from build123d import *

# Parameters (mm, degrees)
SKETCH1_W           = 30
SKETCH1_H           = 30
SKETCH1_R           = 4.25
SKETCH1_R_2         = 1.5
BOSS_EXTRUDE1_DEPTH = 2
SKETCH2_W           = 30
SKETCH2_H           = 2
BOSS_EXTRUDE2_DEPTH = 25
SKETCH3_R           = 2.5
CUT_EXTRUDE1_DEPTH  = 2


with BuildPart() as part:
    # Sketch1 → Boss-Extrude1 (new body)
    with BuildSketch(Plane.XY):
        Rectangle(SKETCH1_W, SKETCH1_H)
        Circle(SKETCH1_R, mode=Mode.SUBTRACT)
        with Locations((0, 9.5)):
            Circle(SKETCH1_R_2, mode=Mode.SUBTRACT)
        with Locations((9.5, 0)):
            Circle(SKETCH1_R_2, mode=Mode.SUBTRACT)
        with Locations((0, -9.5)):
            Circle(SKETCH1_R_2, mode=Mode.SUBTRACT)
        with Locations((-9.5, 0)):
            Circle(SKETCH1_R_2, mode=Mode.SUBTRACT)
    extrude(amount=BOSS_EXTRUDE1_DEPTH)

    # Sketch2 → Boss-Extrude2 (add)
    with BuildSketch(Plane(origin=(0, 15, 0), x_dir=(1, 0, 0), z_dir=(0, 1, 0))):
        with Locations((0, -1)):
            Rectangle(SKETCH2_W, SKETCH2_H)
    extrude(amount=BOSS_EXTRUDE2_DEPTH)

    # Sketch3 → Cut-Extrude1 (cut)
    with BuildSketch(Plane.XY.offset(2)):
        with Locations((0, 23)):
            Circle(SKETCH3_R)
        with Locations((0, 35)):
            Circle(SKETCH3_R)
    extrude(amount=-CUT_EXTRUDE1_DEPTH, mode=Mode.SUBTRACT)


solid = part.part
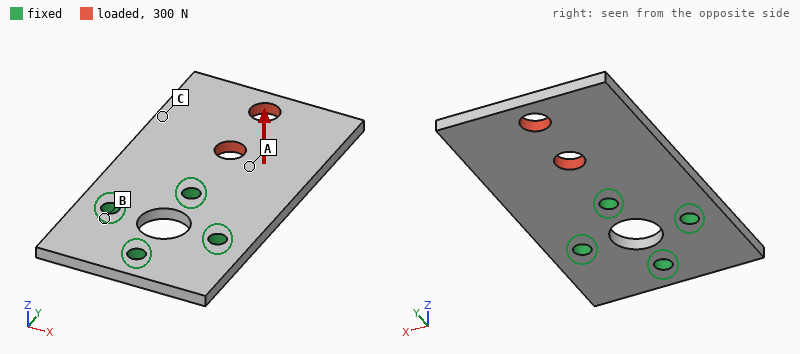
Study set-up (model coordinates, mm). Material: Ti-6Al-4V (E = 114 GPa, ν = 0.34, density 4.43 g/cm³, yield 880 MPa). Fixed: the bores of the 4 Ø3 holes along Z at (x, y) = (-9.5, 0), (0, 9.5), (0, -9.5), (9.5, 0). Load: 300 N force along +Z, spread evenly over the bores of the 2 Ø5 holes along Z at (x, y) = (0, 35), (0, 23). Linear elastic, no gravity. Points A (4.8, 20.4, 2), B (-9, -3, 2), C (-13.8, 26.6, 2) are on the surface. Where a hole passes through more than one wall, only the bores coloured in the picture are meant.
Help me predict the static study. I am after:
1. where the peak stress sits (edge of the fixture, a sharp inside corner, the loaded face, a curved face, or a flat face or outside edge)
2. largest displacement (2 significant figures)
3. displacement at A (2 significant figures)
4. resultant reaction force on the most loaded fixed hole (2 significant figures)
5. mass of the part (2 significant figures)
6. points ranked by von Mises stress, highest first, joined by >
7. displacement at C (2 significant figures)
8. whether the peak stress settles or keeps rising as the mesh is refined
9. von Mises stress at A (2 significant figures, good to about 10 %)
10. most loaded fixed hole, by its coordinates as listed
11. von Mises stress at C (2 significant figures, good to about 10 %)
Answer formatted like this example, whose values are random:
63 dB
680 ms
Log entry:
edge of the fixture
0.70 mm
0.15 mm
560 N
14 g
A > C > B
0.28 mm
keeps rising
140 MPa
(0, 9.5)
79 MPa
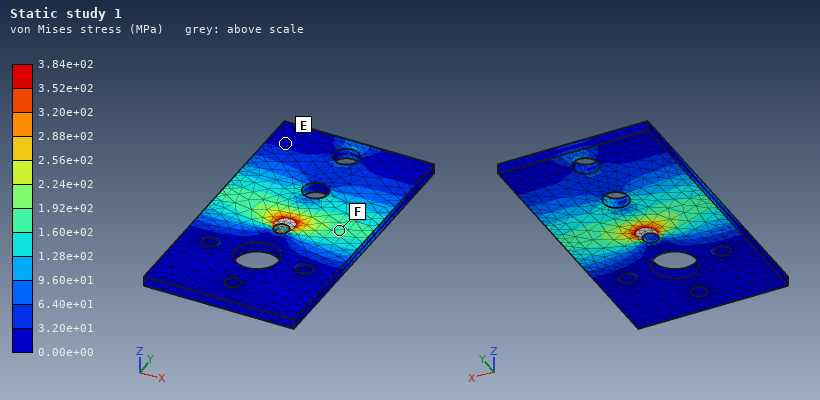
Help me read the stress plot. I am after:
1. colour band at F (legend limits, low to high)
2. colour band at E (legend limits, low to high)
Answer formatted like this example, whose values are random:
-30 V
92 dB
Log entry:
1.60e+02 to 1.92e+02 MPa
0.00e+00 to 3.20e+01 MPa
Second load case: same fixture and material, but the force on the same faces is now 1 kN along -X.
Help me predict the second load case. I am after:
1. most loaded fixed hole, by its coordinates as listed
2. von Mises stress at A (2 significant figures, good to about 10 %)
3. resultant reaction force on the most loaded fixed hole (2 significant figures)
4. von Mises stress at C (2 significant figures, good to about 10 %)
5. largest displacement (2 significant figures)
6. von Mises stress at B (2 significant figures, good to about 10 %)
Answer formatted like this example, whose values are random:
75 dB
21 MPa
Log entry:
(0, 9.5)
36 MPa
1.2 kN
11 MPa
36 µm
14 MPa
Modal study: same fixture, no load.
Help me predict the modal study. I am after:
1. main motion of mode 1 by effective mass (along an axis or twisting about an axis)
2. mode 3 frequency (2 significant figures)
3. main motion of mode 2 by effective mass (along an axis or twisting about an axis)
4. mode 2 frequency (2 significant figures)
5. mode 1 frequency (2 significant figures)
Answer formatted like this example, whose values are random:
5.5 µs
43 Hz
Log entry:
along Z
8500 Hz
twisting about Y
3300 Hz
1700 Hz
